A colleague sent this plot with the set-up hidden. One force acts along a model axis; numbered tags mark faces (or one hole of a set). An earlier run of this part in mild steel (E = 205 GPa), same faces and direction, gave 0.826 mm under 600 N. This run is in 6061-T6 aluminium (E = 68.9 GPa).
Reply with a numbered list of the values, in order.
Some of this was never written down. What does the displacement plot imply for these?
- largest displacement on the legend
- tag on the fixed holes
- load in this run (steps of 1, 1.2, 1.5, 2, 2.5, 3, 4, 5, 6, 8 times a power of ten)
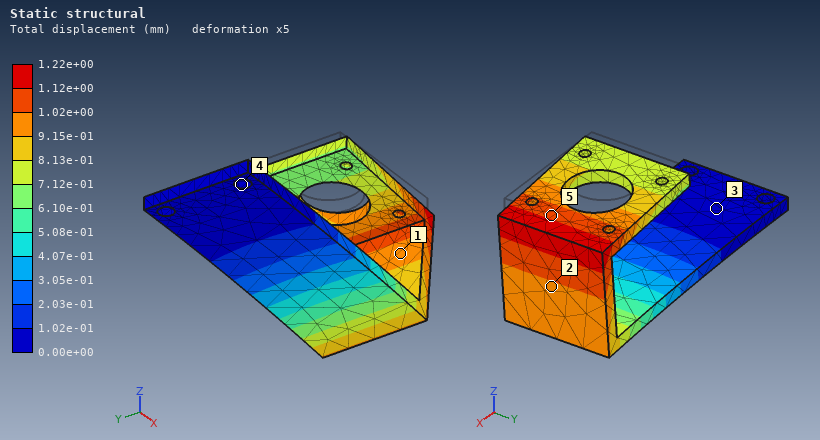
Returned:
1. 1.22e+00 mm
2. 4
3. 300 N
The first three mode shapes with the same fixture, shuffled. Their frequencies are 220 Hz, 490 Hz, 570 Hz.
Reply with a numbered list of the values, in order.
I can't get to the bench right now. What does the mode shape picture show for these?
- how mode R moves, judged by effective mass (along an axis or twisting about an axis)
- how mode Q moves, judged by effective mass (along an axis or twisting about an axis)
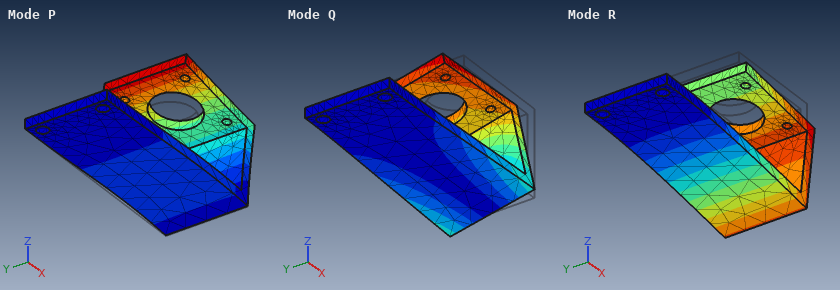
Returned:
1. along Z
2. along Y
